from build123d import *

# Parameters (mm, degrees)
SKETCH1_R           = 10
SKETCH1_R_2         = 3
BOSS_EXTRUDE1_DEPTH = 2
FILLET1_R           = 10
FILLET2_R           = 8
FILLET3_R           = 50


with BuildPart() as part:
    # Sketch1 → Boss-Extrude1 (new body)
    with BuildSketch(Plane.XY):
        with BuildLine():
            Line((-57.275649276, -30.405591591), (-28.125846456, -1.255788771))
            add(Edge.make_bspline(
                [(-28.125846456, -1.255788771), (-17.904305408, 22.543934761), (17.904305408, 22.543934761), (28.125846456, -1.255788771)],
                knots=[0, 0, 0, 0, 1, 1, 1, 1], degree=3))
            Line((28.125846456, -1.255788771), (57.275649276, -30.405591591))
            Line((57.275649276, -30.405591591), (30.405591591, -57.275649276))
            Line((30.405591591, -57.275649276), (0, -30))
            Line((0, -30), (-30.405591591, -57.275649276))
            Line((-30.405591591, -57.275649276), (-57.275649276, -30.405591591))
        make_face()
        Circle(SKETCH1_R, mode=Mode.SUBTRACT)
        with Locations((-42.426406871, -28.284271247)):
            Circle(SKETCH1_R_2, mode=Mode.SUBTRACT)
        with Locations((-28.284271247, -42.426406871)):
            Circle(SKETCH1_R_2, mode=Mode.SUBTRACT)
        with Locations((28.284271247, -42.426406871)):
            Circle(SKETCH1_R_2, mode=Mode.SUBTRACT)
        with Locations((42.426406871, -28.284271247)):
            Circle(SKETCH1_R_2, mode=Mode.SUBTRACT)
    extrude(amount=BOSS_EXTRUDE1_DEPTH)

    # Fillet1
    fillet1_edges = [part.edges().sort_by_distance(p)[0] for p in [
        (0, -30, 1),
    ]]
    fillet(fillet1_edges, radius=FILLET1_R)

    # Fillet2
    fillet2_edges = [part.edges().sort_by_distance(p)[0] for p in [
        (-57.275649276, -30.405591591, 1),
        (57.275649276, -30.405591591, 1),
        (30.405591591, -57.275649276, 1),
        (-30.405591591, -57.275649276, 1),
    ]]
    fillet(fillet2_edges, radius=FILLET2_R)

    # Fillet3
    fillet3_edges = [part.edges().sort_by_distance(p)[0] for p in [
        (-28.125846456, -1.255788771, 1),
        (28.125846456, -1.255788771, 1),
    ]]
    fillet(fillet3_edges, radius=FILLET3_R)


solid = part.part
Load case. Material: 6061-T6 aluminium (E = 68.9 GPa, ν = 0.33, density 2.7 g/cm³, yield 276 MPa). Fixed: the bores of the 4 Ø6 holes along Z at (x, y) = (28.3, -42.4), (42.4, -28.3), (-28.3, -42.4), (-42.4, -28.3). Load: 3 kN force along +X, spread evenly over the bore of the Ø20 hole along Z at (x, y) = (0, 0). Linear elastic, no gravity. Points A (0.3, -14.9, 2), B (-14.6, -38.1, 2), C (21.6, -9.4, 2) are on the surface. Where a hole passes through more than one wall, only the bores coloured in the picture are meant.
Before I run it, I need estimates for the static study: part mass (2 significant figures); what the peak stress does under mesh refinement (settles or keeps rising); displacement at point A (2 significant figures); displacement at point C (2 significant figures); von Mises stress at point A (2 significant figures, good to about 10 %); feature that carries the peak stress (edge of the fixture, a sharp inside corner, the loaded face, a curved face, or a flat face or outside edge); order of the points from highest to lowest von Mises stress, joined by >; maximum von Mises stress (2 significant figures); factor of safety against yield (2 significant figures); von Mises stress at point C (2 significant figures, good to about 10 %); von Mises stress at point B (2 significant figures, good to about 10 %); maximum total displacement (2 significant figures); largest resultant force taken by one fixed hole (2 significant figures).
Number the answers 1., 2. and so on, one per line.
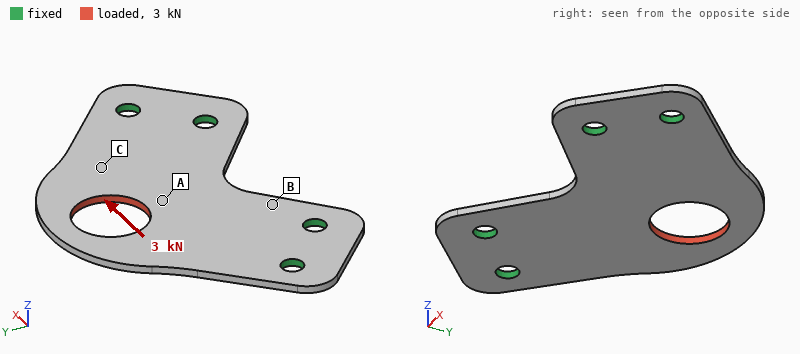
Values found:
1. 23 g
2. settles
3. 16 µm
4. 18 µm
5. 56 MPa
6. the loaded face
7. A > C > B
8. 110 MPa
9. 2.5
10. 28 MPa
11. 15 MPa
12. 56 µm
13. 1.4 kN
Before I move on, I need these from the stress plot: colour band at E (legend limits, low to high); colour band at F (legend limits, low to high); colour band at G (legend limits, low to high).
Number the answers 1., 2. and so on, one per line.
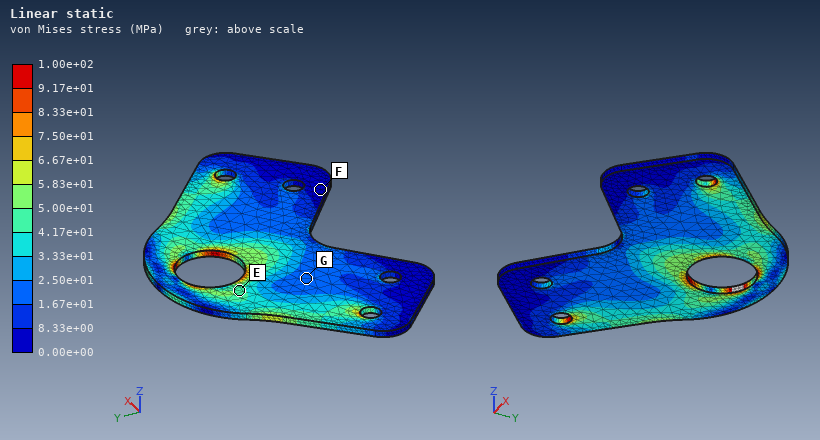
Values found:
1. 4.17e+01 to 5.00e+01 MPa
2. 0.00e+00 to 8.33e+00 MPa
3. 1.67e+01 to 2.50e+01 MPa
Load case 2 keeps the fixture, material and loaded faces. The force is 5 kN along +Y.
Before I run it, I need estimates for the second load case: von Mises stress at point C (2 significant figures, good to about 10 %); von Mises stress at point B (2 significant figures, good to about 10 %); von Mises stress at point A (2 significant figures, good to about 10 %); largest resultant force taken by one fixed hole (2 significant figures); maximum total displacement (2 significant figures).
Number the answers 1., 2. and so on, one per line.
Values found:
1. 44 MPa
2. 37 MPa
3. 35 MPa
4. 2.1 kN
5. 62 µm
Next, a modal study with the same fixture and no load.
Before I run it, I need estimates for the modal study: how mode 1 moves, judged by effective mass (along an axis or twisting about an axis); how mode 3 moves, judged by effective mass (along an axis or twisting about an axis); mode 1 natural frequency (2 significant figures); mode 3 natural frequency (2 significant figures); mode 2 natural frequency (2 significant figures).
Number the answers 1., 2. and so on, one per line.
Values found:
1. along Z
2. along Z
3. 860 Hz
4. 2900 Hz
5. 2300 Hz
